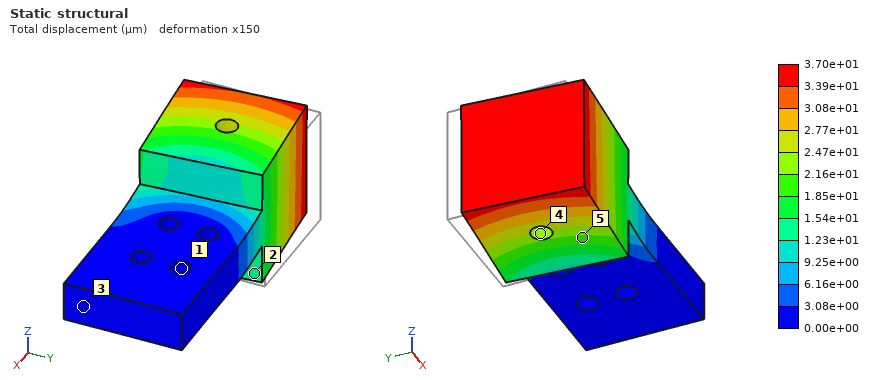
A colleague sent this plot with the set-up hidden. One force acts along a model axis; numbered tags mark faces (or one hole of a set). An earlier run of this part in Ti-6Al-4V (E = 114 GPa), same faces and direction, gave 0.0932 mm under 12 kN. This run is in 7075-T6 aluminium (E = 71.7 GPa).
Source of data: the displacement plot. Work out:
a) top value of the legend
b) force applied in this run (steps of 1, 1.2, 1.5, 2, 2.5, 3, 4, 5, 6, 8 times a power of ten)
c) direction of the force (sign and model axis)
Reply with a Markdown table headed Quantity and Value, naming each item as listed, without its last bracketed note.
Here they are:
| Quantity | Value |
|---|---|
| top value of the legend | 3.70e+01 µm |
| force applied in this run | 3 kN |
| direction of the force | -Y |
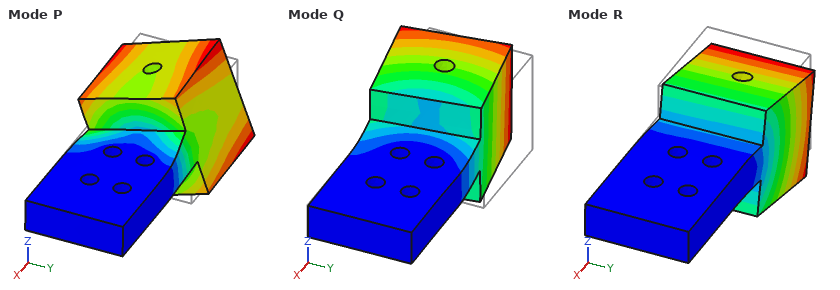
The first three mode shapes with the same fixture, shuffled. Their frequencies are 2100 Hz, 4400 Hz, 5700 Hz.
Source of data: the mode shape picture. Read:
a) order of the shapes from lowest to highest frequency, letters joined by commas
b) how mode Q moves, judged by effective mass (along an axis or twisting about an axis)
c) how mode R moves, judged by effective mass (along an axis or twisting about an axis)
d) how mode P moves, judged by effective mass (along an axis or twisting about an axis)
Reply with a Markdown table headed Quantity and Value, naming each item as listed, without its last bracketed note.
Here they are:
| Quantity | Value |
|---|---|
| order of the shapes from lowest to highest frequency, letters joined by commas | R, Q, P |
| how mode Q moves, judged by effective mass | along Y |
| how mode R moves, judged by effective mass | along Z |
| how mode P moves, judged by effective mass | twisting about X |
